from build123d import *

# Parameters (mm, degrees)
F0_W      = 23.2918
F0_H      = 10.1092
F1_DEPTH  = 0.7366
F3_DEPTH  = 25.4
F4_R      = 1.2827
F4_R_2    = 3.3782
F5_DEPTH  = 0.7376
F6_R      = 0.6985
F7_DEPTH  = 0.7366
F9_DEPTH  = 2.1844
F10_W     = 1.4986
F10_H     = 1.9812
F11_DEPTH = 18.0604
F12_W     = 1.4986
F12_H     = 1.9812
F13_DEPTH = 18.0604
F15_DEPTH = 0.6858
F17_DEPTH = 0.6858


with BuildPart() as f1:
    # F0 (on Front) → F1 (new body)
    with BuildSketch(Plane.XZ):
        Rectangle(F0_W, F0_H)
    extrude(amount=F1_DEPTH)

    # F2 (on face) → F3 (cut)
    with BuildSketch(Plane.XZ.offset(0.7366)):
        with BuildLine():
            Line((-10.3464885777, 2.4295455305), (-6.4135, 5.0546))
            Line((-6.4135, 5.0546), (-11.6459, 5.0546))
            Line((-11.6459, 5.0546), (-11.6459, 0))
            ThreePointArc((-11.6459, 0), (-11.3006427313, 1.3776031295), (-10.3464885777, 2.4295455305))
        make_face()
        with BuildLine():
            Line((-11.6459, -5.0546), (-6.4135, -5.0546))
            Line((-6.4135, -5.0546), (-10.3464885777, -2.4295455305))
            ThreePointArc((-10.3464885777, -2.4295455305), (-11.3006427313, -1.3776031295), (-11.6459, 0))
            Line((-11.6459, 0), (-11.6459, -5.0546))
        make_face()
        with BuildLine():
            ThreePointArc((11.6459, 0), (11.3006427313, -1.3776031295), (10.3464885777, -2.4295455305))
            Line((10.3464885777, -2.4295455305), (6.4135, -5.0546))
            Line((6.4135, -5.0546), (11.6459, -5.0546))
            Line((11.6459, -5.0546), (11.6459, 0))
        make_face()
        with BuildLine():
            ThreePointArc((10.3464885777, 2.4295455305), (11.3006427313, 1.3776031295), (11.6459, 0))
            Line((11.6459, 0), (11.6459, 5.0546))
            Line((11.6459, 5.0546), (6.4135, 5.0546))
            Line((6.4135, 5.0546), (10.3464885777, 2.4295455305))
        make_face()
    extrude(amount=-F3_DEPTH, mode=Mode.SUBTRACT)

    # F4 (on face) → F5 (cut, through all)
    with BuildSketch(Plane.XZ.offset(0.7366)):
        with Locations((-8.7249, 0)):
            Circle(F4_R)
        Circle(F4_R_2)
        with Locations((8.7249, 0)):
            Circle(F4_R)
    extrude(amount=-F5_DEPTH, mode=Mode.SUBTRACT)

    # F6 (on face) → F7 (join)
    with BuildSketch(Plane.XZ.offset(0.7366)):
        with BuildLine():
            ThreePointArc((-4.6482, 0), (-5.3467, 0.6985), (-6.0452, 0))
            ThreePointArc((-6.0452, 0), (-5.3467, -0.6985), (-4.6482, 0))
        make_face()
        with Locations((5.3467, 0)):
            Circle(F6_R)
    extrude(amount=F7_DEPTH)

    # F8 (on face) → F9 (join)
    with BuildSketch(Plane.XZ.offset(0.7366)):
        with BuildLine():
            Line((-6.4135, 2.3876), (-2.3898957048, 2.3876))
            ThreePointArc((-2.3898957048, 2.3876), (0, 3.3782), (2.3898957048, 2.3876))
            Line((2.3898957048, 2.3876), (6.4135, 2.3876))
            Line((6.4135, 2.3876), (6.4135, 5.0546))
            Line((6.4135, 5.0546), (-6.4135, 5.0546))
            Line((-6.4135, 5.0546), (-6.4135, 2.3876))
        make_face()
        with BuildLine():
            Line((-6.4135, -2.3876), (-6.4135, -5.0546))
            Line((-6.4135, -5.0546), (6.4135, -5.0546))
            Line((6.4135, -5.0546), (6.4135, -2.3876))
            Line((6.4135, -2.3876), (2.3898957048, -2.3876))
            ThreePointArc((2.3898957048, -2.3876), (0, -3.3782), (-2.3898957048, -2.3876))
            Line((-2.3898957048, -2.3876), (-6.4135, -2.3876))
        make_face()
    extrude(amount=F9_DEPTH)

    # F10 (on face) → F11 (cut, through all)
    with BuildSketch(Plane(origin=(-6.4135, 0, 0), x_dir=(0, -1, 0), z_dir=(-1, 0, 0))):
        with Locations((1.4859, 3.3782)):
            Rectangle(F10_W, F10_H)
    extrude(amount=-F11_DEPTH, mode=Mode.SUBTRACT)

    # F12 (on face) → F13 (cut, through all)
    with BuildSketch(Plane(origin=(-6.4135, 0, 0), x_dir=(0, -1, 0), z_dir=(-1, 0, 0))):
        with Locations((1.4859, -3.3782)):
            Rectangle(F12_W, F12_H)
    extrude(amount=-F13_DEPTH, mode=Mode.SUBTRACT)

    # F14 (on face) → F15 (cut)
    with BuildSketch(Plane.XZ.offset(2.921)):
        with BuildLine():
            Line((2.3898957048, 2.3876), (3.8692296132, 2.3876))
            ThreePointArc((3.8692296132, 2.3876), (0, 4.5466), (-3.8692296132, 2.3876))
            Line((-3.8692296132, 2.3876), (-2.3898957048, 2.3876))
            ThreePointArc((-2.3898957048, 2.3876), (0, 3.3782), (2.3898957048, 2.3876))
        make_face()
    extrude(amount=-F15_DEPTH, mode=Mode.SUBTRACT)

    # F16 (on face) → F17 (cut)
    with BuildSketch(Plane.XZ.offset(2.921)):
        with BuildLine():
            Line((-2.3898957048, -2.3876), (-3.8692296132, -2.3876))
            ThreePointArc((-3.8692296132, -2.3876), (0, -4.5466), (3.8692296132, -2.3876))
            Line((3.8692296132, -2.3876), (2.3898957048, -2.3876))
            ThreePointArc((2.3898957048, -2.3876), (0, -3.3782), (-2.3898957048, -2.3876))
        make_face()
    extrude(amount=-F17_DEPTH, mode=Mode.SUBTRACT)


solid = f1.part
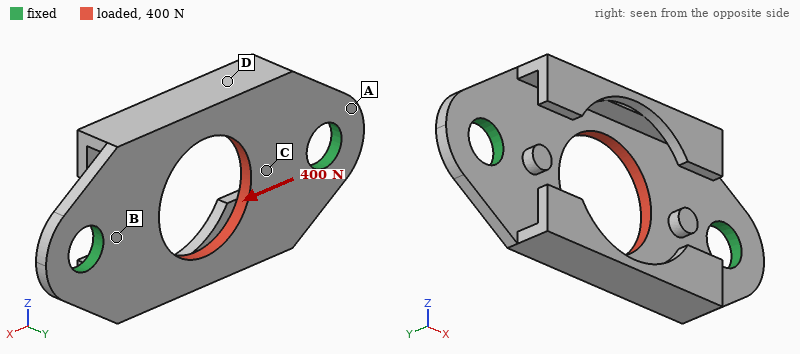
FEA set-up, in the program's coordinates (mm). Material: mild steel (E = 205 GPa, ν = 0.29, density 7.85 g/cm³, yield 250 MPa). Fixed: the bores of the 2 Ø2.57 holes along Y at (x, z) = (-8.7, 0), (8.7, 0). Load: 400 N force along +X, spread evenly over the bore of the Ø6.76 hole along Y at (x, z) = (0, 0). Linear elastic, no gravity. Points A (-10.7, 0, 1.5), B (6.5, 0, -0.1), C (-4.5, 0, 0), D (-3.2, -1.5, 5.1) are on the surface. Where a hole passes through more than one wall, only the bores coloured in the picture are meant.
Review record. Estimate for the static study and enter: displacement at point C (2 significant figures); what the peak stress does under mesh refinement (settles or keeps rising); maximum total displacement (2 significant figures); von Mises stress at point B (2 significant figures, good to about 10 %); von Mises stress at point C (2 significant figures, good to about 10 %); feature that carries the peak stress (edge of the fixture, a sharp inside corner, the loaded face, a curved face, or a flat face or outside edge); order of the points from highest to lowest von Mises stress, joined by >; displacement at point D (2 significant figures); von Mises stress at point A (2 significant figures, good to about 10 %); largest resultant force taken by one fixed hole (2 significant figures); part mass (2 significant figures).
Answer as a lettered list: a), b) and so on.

a) 0.65 µm
b) keeps rising
c) 1.6 µm
d) 52 MPa
e) 39 MPa
f) edge of the fixture
g) B > C > A > D
h) 1.2 µm
i) 17 MPa
j) 200 N
k) 1.3 g
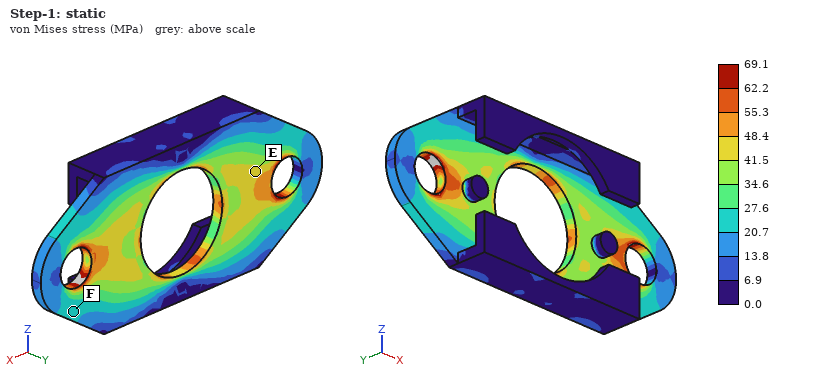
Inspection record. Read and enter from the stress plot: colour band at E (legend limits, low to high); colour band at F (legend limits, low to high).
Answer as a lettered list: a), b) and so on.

a) 41.5 to 48.4 MPa
b) 20.7 to 27.6 MPa
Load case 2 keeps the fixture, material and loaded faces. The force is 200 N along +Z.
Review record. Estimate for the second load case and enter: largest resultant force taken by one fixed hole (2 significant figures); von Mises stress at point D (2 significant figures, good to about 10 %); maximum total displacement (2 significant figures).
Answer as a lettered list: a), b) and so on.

a) 100 N
b) 9.2 MPa
c) 3.5 µm
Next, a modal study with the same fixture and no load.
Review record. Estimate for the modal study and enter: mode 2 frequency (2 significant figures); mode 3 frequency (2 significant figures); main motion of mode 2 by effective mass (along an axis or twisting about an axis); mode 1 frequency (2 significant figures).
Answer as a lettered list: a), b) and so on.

a) 14 kHz
b) 24 kHz
c) along Y
d) 12 kHz
